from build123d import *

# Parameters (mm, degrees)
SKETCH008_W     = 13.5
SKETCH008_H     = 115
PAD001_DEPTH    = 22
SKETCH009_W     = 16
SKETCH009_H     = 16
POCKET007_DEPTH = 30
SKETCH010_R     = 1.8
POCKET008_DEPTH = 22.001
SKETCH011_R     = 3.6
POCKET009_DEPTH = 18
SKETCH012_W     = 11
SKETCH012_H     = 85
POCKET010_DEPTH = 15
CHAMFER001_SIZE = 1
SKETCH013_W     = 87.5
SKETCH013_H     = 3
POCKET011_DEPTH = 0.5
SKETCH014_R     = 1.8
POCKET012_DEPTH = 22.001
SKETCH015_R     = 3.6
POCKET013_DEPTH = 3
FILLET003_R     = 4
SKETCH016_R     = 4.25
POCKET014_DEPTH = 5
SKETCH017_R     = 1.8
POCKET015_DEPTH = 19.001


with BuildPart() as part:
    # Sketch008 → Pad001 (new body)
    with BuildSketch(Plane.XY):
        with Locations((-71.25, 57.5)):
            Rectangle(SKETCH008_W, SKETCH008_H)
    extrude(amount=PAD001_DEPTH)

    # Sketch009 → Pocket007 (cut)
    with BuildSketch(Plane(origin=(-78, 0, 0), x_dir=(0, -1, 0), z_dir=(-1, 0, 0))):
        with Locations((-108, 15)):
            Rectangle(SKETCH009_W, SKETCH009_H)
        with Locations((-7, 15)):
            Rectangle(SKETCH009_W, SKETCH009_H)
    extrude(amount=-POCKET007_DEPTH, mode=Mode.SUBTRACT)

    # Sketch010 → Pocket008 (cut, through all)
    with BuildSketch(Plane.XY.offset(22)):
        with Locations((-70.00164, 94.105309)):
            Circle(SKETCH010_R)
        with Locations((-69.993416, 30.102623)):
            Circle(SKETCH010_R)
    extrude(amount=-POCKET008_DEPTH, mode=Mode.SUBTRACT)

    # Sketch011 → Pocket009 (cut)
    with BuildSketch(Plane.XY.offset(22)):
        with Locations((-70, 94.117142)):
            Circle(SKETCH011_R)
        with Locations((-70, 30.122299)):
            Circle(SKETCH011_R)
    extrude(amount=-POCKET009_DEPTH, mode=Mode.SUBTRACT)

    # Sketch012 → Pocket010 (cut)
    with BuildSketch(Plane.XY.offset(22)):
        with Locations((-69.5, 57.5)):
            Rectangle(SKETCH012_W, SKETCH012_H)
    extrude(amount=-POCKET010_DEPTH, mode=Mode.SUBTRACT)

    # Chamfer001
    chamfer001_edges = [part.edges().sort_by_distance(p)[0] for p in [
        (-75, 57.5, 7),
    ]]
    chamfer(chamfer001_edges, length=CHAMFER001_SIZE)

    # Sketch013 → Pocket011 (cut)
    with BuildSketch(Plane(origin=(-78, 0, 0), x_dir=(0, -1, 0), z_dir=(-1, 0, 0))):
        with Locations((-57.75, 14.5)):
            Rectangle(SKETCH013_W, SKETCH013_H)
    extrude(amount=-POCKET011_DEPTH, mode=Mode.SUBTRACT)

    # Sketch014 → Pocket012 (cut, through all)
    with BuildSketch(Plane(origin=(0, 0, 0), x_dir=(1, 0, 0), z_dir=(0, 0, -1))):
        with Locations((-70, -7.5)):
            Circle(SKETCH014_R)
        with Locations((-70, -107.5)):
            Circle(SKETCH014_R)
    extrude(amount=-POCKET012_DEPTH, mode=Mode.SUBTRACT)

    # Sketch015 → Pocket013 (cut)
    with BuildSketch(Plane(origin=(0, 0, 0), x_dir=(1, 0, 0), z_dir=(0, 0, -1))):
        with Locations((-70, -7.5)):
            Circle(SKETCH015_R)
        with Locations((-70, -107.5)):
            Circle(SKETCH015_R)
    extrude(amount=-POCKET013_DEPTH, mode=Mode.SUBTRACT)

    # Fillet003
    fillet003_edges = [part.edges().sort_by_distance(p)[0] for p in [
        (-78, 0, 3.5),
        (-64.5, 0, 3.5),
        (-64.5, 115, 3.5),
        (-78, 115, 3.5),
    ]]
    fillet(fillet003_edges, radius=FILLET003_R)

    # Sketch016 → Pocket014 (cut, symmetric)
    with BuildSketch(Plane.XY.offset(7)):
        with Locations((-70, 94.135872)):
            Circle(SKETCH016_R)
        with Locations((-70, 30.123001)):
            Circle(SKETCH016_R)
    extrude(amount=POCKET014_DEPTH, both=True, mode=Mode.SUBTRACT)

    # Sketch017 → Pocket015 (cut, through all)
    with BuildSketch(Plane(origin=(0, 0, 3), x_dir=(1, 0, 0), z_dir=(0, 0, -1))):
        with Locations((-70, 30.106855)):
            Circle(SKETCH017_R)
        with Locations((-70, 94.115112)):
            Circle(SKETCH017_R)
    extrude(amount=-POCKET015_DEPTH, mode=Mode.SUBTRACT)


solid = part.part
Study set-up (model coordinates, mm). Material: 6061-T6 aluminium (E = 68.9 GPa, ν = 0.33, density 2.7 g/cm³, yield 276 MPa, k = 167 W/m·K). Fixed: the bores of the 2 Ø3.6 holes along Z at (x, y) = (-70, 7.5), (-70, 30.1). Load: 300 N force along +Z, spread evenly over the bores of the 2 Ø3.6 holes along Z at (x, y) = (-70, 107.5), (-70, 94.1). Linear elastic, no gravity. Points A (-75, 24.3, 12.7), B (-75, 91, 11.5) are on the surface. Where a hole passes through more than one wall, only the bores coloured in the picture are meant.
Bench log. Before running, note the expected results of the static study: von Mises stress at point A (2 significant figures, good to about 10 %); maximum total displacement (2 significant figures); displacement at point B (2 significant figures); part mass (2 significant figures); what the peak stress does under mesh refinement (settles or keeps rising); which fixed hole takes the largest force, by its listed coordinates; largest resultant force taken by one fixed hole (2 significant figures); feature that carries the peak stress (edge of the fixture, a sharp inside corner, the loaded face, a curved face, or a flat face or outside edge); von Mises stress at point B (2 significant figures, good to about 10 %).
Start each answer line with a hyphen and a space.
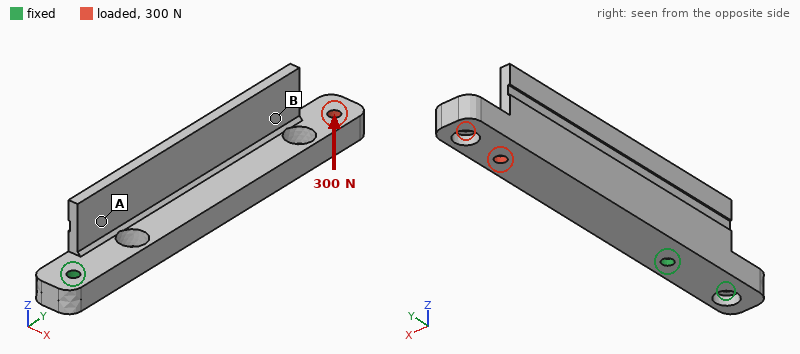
- 57 MPa
- 0.57 mm
- 0.36 mm
- 37 g
- keeps rising
- (-70, 30.1)
- 1.4 kN
- edge of the fixture
- 20 MPa
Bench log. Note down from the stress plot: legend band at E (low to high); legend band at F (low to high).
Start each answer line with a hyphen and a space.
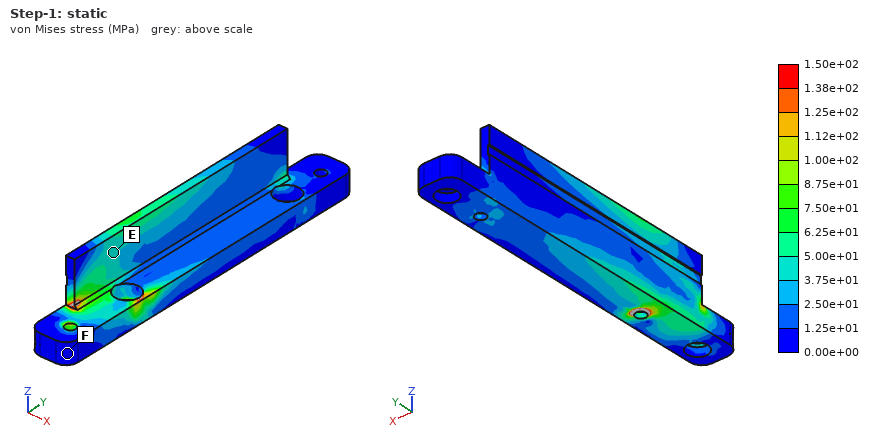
- 3.75e+01 to 5.00e+01 MPa
- 0.00e+00 to 1.25e+01 MPa
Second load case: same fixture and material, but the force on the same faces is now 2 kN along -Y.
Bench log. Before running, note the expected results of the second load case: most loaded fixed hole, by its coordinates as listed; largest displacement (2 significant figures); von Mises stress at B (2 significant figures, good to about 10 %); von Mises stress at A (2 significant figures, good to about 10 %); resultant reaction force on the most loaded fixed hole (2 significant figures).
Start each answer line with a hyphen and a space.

- (-70, 30.1)
- 0.16 mm
- 12 MPa
- 9.7 MPa
- 1.4 kN
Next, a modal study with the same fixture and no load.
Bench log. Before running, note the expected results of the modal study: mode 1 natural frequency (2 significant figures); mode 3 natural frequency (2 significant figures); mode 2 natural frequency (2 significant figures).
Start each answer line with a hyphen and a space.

- 1100 Hz
- 3200 Hz
- 1600 Hz
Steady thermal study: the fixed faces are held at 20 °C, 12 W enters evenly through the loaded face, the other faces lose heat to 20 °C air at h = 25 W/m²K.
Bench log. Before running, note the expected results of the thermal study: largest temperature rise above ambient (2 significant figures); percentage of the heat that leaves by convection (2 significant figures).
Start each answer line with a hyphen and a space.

- 43 K
- 27 %
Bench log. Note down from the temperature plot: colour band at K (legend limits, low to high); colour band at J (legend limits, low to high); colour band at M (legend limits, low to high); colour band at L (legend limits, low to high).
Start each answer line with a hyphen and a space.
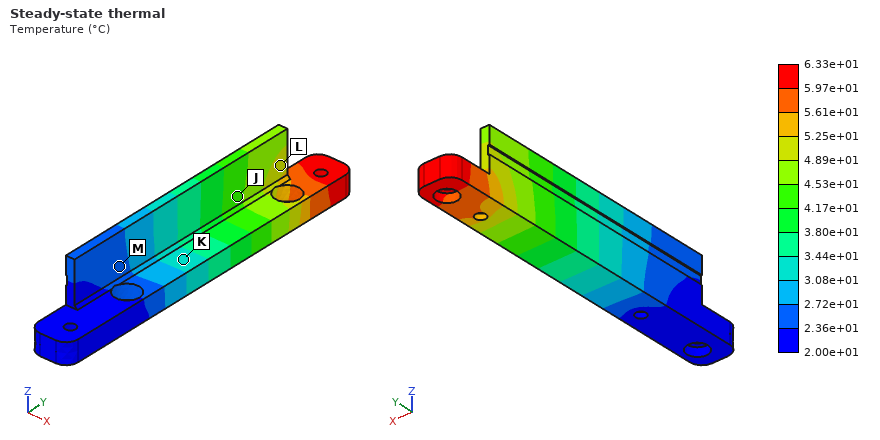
- 3.08e+01 to 3.44e+01 °C
- 4.17e+01 to 4.53e+01 °C
- 2.36e+01 to 2.72e+01 °C
- 4.89e+01 to 5.25e+01 °C
